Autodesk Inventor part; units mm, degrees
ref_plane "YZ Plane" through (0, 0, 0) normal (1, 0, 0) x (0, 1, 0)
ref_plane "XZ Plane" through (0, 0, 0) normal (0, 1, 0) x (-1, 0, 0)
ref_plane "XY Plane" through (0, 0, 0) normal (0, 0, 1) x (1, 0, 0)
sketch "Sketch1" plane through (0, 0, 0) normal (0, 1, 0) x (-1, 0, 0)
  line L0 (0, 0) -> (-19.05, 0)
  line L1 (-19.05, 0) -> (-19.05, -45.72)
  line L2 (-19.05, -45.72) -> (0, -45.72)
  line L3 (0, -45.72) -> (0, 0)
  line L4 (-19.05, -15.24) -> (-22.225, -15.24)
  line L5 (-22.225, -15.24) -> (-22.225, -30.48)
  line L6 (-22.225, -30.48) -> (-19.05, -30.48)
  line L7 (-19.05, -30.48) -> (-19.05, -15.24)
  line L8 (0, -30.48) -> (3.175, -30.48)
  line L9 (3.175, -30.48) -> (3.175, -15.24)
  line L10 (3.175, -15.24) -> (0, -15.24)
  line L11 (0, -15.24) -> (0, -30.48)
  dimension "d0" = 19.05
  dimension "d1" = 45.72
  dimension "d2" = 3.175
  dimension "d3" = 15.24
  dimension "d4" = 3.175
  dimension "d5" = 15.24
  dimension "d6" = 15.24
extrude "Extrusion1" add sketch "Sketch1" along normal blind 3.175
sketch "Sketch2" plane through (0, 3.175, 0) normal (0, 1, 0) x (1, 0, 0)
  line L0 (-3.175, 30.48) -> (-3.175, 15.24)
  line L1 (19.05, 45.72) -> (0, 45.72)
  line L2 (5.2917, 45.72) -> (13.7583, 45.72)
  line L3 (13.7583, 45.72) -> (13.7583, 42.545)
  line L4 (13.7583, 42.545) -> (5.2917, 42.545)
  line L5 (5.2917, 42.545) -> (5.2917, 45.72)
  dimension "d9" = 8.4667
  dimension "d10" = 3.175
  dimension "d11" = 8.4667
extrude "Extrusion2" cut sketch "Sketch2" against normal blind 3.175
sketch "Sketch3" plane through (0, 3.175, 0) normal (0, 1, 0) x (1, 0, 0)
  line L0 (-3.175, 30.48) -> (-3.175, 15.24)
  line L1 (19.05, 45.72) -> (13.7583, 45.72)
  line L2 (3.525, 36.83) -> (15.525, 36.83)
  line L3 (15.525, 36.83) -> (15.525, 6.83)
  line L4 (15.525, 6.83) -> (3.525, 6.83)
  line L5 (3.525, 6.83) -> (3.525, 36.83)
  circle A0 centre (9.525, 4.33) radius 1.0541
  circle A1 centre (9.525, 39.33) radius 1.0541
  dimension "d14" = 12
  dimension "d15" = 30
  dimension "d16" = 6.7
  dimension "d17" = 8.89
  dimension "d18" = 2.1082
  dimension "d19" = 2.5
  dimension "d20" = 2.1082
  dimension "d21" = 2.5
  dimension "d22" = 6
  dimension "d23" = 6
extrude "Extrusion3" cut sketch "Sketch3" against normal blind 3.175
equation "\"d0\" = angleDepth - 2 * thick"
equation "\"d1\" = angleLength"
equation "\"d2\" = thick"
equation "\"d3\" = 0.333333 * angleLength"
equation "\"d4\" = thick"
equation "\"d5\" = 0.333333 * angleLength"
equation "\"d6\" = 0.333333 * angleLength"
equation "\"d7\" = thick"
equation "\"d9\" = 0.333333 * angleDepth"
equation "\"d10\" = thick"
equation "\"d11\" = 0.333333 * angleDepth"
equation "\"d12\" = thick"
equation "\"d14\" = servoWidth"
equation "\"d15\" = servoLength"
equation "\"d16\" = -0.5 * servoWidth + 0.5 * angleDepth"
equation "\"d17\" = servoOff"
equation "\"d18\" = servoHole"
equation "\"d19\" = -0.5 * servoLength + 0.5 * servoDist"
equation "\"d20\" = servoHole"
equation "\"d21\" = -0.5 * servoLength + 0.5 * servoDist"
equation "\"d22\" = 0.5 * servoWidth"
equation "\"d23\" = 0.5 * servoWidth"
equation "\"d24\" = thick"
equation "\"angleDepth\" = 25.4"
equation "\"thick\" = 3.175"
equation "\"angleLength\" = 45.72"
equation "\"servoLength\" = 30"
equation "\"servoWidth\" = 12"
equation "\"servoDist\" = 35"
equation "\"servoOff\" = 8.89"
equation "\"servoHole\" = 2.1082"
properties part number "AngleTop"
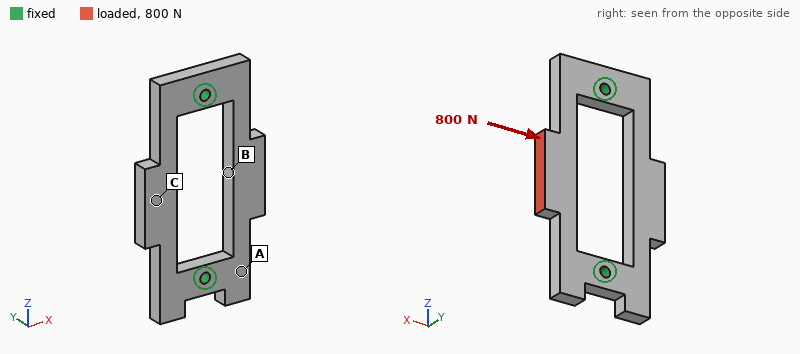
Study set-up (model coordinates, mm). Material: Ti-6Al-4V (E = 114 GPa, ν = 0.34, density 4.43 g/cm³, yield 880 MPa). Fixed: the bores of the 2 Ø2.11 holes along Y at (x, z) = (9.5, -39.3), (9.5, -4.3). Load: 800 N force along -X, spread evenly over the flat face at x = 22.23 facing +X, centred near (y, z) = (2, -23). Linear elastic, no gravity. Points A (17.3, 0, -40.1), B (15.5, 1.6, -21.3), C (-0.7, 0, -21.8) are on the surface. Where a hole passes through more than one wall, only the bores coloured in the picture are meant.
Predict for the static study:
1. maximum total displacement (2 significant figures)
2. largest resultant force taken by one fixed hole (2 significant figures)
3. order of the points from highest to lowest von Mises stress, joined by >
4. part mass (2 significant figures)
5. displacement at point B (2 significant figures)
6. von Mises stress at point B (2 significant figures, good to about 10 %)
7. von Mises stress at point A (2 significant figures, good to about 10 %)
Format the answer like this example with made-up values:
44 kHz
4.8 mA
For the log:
54 µm
570 N
B > A > C
8.1 g
54 µm
86 MPa
55 MPa
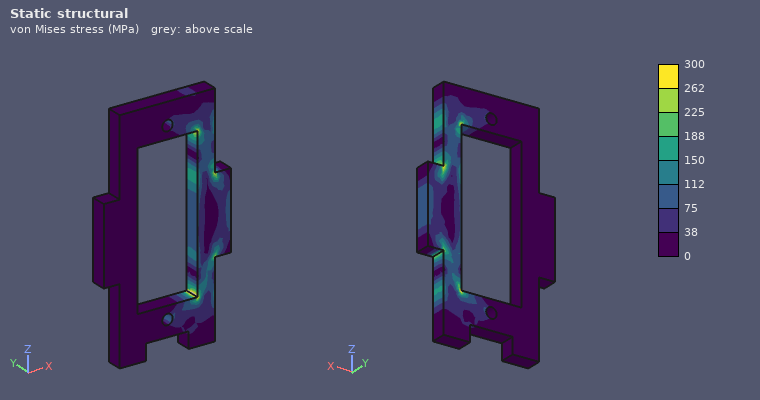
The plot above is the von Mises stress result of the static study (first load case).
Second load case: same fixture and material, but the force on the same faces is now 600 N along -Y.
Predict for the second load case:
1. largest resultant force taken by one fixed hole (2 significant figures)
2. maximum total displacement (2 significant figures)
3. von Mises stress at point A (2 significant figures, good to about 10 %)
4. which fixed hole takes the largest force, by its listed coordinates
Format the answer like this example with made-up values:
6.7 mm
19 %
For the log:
320 N
0.34 mm
190 MPa
(9.5, -39.3)
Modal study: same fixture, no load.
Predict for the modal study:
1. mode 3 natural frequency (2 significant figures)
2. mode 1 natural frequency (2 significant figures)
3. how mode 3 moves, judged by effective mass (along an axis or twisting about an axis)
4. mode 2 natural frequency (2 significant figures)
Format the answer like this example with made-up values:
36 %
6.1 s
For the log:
15 kHz
7100 Hz
along X
7100 Hz
